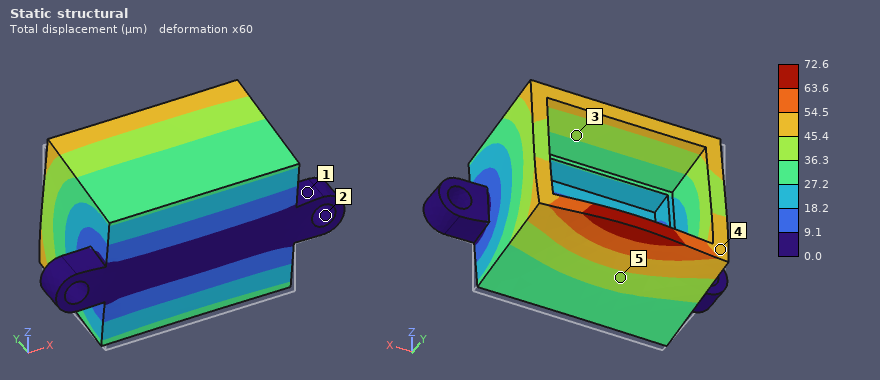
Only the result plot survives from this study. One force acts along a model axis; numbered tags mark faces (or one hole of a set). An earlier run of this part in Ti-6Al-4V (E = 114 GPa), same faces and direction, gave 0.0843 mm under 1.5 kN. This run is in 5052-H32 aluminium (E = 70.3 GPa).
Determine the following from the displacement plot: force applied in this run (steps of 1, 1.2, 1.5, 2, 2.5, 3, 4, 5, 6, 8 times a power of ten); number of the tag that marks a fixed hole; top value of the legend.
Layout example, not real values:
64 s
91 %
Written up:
800 N
2
72.6 µm
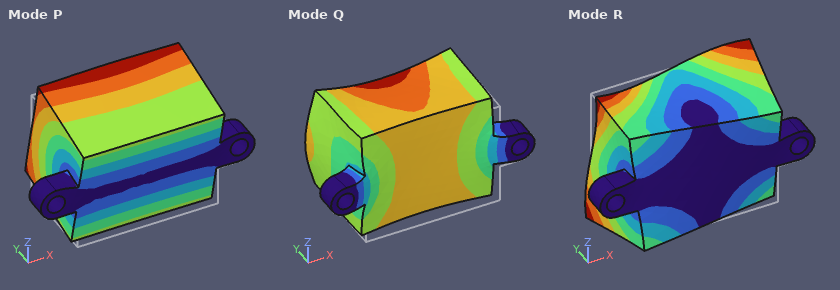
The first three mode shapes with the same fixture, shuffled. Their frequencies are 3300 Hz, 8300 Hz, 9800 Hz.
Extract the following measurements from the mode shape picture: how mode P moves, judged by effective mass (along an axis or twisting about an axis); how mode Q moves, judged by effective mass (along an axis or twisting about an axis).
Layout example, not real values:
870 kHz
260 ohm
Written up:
along Z
along Y
